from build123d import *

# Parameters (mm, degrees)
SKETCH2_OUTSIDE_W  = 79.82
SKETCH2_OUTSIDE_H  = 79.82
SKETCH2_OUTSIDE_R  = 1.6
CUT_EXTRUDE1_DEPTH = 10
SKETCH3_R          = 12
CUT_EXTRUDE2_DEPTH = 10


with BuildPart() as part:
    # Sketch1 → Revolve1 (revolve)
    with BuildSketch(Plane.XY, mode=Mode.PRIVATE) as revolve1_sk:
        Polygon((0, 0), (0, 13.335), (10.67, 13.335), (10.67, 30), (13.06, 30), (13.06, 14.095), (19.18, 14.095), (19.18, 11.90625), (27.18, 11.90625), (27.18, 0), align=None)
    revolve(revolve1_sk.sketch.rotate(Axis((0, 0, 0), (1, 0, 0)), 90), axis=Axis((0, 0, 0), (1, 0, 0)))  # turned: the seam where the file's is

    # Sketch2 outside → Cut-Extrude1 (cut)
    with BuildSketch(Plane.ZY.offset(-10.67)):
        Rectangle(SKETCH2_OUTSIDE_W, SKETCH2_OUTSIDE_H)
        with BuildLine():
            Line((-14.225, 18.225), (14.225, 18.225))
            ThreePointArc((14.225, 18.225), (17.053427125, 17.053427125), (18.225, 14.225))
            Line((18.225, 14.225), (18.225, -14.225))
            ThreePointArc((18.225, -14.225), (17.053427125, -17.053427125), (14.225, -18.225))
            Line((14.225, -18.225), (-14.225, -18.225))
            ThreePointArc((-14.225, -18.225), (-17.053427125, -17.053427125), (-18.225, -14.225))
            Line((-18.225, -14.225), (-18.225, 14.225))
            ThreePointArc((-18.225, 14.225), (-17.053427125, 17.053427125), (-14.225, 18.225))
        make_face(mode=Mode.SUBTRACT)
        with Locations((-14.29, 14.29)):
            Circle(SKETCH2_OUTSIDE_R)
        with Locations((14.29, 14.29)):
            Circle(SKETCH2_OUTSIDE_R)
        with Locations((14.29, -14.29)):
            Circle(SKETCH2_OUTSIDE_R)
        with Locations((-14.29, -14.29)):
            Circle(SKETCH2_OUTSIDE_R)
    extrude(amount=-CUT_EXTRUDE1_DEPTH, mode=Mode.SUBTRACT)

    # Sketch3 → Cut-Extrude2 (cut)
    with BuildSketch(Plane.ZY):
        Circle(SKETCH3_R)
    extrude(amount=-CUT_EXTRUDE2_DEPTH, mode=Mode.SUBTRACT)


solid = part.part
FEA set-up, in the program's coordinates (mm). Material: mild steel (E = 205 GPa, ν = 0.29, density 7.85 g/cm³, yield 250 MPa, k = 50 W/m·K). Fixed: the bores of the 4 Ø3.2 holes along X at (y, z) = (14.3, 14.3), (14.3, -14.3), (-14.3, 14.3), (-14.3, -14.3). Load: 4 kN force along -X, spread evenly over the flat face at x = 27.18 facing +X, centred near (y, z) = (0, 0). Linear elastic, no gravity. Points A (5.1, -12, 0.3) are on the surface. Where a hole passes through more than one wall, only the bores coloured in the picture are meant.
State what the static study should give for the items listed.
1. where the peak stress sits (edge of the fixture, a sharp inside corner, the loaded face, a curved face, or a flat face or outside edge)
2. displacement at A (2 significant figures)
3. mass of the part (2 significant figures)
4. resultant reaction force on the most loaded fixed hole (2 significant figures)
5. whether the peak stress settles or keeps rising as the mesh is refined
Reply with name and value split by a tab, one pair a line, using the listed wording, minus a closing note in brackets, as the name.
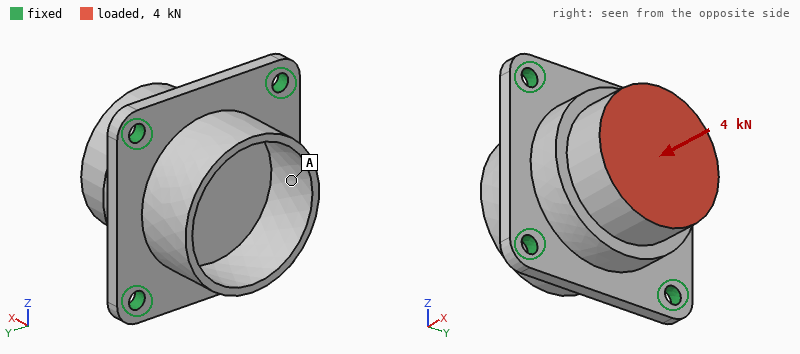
where the peak stress sits	edge of the fixture
displacement at A	13 µm
mass of the part	93 g
resultant reaction force on the most loaded fixed hole	1.0 kN
whether the peak stress settles or keeps rising as the mesh is refined	keeps rising
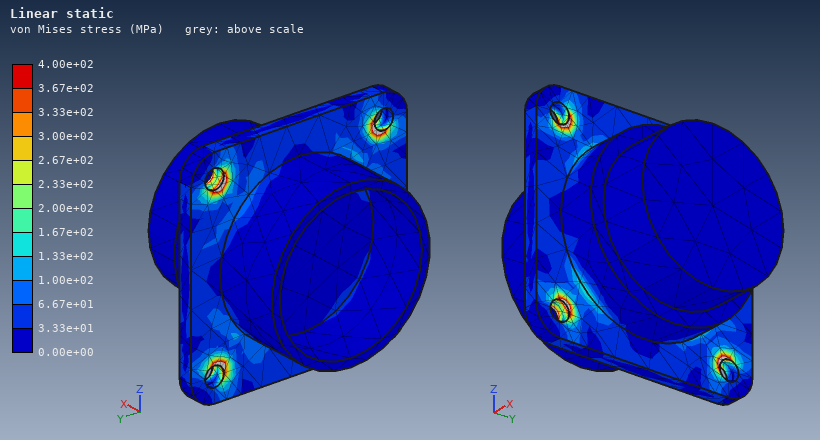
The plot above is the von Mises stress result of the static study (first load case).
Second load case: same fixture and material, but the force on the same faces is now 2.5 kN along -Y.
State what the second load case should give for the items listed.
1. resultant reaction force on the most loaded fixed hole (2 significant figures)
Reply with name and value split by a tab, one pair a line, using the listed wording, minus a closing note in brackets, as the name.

resultant reaction force on the most loaded fixed hole	1.0 kN
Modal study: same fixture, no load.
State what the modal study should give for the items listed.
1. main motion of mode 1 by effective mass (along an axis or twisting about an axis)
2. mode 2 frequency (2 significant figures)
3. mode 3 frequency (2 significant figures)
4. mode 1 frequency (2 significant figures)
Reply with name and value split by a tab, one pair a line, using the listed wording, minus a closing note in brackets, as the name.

main motion of mode 1 by effective mass	along X
mode 2 frequency	11 kHz
mode 3 frequency	11 kHz
mode 1 frequency	9400 Hz
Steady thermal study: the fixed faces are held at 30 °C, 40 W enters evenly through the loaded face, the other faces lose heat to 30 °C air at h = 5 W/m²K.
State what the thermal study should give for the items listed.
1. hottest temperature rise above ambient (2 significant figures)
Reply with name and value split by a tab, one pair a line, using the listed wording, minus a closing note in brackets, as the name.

hottest temperature rise above ambient	73 K
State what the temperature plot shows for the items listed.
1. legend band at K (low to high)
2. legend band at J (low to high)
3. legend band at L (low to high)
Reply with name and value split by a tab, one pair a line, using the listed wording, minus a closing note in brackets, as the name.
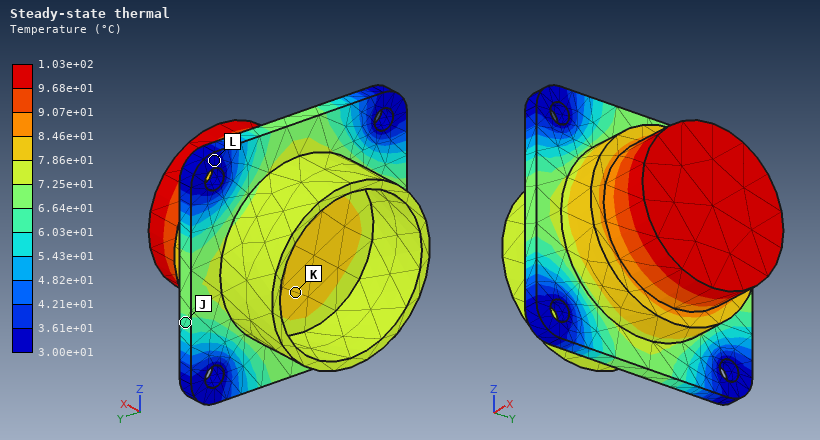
legend band at K	7.86e+01 to 8.46e+01 °C
legend band at J	6.03e+01 to 6.64e+01 °C
legend band at L	3.00e+01 to 3.61e+01 °C
